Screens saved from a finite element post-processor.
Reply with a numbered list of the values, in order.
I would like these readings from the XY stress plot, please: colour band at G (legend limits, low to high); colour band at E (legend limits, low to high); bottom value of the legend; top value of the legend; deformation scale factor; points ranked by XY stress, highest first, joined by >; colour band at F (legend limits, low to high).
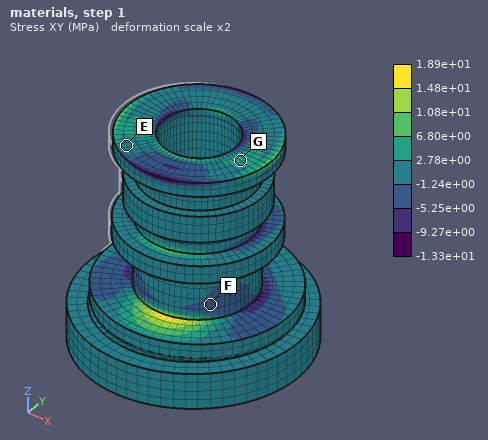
1. 2.78e+00 to 6.80e+00 MPa
2. -1.24e+00 to 2.78e+00 MPa
3. -1.33e+01 MPa
4. 1.89e+01 MPa
5. 2
6. G > E > F
7. -5.25e+00 to -1.24e+00 MPa
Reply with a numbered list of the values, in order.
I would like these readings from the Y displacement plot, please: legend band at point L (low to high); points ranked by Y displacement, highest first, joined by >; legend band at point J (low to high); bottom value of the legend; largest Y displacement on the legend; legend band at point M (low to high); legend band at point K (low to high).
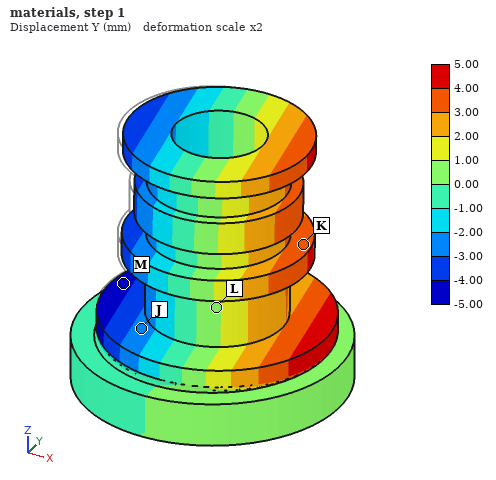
1. 0.00 to 1.00 mm
2. K > L > J > M
3. -3.00 to -2.00 mm
4. -5.00 mm
5. 5.00 mm
6. -5.00 to -4.00 mm
7. 3.00 to 4.00 mm
